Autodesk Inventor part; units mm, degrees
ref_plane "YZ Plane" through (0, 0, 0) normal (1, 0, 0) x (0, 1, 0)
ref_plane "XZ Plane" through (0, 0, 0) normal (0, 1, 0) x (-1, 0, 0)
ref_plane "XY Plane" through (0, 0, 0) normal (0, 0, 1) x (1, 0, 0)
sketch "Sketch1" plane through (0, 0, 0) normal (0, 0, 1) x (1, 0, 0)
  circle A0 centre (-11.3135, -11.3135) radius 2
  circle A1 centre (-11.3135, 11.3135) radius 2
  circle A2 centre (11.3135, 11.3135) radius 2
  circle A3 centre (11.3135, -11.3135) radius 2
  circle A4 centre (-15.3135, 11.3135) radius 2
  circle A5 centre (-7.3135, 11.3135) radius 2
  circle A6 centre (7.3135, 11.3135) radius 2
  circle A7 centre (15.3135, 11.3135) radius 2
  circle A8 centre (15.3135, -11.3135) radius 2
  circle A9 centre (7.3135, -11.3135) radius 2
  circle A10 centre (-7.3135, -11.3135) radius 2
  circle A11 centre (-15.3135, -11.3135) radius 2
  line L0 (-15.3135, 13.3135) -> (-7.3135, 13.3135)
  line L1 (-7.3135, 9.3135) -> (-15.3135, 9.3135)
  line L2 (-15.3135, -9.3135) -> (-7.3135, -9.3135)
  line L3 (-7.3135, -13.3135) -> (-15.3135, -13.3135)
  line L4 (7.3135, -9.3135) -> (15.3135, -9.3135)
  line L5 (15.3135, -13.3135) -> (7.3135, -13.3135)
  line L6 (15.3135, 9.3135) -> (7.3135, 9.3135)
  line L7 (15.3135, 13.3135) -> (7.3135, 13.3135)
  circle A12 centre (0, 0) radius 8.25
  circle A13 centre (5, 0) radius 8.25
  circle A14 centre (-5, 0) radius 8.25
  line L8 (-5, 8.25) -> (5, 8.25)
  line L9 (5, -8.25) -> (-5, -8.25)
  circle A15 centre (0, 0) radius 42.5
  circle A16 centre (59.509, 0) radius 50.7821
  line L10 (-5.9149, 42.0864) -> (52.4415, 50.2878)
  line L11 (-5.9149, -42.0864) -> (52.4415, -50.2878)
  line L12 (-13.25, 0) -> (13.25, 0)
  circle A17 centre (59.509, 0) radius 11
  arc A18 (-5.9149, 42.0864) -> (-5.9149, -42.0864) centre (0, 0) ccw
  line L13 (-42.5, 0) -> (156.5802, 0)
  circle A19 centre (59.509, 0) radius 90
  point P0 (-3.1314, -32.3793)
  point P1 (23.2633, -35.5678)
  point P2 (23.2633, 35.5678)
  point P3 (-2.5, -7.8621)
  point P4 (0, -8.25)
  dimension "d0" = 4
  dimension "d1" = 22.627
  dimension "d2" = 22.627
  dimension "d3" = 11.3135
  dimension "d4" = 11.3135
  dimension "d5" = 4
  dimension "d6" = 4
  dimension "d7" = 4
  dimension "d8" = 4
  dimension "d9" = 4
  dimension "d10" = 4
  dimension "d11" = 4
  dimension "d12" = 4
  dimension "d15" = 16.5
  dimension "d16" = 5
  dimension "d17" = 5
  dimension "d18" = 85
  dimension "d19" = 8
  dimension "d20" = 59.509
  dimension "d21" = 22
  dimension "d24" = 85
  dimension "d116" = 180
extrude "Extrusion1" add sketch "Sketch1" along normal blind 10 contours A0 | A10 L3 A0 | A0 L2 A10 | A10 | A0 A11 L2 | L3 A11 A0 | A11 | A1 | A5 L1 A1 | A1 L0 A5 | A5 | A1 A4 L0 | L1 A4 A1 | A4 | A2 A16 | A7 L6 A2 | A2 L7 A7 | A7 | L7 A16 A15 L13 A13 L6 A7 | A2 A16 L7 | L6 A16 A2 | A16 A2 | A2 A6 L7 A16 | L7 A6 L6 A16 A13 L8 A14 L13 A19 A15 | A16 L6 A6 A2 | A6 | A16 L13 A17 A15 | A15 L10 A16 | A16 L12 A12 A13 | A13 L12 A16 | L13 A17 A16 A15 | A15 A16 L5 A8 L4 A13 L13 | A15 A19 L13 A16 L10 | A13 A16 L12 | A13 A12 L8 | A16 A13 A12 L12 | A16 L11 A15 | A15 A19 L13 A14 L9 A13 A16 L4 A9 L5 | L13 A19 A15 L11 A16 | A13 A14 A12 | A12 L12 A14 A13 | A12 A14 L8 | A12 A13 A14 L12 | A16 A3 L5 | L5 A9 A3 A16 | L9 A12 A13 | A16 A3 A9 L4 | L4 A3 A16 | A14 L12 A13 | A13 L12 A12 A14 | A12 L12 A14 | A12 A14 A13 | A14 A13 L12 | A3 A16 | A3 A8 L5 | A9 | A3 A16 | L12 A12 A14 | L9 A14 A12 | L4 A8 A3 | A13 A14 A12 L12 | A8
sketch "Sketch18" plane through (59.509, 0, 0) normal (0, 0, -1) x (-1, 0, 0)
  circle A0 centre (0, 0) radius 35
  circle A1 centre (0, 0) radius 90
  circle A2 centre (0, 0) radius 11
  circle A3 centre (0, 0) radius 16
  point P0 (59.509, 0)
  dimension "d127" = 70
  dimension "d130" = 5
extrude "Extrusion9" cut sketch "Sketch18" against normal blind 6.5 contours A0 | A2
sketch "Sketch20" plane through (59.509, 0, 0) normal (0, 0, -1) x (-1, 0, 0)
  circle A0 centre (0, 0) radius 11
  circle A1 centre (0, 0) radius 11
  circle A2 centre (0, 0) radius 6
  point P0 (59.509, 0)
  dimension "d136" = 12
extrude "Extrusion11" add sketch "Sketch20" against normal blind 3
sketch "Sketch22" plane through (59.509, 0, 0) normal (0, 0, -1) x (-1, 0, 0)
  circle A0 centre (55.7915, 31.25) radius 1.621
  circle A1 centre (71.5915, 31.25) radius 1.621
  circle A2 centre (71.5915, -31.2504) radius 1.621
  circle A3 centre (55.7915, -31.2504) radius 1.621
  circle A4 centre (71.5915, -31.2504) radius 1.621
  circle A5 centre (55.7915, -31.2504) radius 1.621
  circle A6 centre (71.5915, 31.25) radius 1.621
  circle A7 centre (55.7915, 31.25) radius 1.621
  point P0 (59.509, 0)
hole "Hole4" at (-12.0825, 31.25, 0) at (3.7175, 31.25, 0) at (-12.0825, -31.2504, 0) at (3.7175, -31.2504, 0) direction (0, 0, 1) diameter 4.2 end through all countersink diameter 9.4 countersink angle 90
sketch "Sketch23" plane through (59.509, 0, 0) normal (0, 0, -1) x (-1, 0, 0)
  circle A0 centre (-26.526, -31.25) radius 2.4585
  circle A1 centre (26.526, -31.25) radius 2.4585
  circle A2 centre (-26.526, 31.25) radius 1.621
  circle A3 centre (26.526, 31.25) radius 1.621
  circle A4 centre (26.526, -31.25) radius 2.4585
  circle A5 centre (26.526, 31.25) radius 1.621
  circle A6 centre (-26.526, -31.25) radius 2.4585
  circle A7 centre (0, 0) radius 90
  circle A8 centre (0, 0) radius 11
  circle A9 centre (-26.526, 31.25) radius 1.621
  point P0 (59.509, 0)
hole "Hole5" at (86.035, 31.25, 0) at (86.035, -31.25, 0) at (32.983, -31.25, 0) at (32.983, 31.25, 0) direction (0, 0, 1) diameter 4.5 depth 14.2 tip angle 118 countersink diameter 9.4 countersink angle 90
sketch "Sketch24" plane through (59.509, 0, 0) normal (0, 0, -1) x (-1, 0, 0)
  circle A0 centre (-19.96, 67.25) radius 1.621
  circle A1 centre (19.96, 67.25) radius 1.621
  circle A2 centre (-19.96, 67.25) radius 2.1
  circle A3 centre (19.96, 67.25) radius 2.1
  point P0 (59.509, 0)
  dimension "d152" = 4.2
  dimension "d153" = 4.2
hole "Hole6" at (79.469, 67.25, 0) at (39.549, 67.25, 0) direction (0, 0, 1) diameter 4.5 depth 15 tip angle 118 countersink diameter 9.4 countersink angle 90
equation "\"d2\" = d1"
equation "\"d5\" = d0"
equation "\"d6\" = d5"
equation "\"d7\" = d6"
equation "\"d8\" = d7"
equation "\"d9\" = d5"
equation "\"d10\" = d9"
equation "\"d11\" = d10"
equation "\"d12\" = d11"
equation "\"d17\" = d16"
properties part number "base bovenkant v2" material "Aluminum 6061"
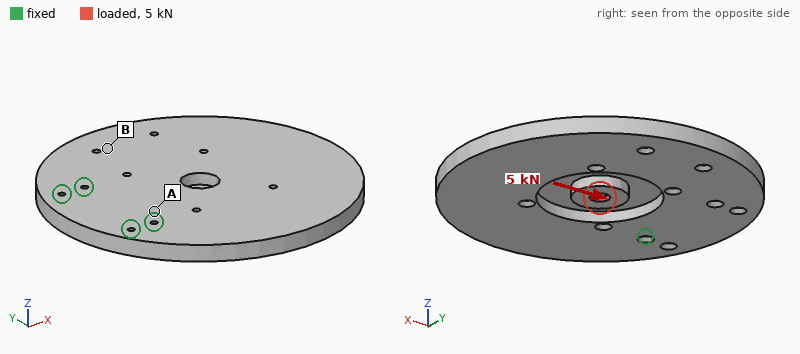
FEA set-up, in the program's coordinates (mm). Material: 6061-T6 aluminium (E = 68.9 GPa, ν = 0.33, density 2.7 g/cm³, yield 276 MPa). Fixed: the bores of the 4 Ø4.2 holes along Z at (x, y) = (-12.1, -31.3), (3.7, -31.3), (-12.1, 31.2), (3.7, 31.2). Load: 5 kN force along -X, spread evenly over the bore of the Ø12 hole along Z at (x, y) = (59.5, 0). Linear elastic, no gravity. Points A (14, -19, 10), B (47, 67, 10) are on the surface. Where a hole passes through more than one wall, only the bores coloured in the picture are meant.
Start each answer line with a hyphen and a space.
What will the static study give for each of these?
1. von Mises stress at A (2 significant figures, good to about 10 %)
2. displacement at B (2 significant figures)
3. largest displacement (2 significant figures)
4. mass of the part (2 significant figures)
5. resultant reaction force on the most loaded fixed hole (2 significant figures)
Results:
- 13 MPa
- 0.054 mm
- 0.29 mm
- 620 g
- 1.6 kN
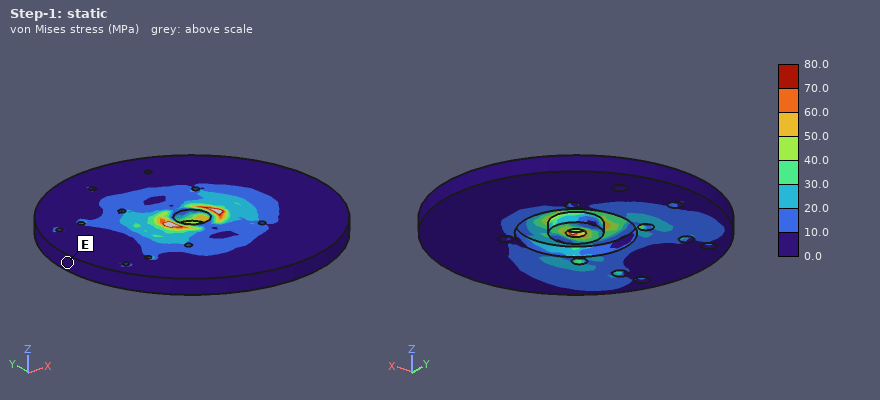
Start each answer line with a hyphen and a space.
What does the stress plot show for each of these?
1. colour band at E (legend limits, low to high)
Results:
- 0.0 to 10.0 MPa
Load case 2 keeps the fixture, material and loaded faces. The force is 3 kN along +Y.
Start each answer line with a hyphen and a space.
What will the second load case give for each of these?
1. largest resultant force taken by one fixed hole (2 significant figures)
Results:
- 2.4 kN
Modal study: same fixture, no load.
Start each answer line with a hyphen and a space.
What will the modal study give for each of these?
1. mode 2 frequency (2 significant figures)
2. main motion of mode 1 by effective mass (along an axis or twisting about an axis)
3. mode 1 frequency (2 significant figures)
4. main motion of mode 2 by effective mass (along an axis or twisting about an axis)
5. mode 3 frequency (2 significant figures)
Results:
- 750 Hz
- along Z
- 360 Hz
- twisting about X
- 1600 Hz
